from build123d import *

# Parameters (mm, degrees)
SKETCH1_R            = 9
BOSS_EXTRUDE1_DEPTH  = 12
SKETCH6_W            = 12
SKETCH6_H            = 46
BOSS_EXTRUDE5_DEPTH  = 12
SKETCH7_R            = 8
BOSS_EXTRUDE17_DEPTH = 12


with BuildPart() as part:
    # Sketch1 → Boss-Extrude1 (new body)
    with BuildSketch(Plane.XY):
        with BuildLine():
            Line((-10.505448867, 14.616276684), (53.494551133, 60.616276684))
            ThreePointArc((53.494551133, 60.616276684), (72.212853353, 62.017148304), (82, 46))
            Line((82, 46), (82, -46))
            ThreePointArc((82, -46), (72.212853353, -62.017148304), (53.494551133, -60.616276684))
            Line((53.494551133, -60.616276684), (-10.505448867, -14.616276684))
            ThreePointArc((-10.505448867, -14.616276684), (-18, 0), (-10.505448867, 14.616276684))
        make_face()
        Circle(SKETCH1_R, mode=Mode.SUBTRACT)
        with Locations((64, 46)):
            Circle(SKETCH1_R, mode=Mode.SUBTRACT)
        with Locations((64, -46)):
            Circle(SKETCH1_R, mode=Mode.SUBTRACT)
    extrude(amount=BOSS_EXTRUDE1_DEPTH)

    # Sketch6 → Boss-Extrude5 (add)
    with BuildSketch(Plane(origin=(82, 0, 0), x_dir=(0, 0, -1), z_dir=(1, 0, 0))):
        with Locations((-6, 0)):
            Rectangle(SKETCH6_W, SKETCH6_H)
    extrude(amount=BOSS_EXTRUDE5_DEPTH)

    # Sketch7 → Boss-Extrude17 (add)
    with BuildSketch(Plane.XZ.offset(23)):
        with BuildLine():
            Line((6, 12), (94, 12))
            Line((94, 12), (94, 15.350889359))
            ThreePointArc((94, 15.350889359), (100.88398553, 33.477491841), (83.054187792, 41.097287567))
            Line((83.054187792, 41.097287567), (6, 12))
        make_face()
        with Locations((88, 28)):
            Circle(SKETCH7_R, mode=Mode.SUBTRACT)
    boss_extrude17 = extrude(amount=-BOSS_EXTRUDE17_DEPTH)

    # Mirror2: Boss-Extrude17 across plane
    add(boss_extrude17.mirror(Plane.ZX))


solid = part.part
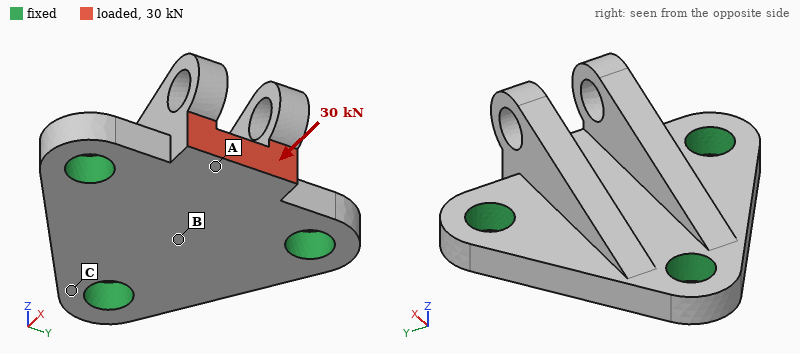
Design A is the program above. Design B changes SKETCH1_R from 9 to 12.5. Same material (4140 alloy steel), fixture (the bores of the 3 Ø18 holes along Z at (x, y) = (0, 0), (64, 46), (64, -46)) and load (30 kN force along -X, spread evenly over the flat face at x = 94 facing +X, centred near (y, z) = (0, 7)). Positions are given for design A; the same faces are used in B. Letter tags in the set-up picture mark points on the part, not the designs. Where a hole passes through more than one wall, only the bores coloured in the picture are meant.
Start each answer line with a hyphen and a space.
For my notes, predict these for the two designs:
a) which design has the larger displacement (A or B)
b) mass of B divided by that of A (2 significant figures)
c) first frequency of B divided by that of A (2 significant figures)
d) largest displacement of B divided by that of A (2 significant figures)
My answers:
- A
- 0.94
- 1.1
- 0.91
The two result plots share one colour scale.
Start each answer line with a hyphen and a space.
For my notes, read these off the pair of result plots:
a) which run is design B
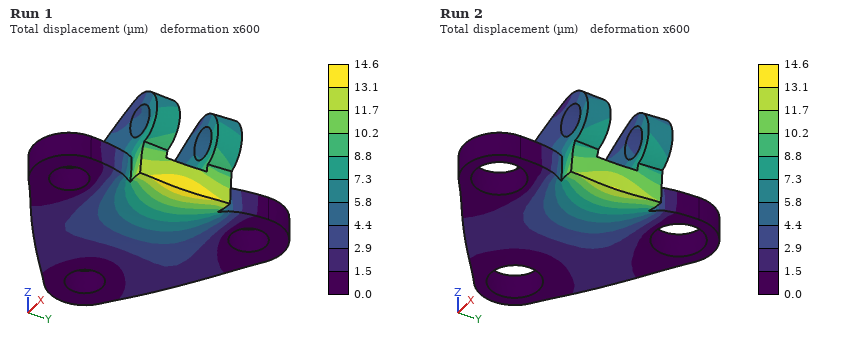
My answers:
- Run 2
